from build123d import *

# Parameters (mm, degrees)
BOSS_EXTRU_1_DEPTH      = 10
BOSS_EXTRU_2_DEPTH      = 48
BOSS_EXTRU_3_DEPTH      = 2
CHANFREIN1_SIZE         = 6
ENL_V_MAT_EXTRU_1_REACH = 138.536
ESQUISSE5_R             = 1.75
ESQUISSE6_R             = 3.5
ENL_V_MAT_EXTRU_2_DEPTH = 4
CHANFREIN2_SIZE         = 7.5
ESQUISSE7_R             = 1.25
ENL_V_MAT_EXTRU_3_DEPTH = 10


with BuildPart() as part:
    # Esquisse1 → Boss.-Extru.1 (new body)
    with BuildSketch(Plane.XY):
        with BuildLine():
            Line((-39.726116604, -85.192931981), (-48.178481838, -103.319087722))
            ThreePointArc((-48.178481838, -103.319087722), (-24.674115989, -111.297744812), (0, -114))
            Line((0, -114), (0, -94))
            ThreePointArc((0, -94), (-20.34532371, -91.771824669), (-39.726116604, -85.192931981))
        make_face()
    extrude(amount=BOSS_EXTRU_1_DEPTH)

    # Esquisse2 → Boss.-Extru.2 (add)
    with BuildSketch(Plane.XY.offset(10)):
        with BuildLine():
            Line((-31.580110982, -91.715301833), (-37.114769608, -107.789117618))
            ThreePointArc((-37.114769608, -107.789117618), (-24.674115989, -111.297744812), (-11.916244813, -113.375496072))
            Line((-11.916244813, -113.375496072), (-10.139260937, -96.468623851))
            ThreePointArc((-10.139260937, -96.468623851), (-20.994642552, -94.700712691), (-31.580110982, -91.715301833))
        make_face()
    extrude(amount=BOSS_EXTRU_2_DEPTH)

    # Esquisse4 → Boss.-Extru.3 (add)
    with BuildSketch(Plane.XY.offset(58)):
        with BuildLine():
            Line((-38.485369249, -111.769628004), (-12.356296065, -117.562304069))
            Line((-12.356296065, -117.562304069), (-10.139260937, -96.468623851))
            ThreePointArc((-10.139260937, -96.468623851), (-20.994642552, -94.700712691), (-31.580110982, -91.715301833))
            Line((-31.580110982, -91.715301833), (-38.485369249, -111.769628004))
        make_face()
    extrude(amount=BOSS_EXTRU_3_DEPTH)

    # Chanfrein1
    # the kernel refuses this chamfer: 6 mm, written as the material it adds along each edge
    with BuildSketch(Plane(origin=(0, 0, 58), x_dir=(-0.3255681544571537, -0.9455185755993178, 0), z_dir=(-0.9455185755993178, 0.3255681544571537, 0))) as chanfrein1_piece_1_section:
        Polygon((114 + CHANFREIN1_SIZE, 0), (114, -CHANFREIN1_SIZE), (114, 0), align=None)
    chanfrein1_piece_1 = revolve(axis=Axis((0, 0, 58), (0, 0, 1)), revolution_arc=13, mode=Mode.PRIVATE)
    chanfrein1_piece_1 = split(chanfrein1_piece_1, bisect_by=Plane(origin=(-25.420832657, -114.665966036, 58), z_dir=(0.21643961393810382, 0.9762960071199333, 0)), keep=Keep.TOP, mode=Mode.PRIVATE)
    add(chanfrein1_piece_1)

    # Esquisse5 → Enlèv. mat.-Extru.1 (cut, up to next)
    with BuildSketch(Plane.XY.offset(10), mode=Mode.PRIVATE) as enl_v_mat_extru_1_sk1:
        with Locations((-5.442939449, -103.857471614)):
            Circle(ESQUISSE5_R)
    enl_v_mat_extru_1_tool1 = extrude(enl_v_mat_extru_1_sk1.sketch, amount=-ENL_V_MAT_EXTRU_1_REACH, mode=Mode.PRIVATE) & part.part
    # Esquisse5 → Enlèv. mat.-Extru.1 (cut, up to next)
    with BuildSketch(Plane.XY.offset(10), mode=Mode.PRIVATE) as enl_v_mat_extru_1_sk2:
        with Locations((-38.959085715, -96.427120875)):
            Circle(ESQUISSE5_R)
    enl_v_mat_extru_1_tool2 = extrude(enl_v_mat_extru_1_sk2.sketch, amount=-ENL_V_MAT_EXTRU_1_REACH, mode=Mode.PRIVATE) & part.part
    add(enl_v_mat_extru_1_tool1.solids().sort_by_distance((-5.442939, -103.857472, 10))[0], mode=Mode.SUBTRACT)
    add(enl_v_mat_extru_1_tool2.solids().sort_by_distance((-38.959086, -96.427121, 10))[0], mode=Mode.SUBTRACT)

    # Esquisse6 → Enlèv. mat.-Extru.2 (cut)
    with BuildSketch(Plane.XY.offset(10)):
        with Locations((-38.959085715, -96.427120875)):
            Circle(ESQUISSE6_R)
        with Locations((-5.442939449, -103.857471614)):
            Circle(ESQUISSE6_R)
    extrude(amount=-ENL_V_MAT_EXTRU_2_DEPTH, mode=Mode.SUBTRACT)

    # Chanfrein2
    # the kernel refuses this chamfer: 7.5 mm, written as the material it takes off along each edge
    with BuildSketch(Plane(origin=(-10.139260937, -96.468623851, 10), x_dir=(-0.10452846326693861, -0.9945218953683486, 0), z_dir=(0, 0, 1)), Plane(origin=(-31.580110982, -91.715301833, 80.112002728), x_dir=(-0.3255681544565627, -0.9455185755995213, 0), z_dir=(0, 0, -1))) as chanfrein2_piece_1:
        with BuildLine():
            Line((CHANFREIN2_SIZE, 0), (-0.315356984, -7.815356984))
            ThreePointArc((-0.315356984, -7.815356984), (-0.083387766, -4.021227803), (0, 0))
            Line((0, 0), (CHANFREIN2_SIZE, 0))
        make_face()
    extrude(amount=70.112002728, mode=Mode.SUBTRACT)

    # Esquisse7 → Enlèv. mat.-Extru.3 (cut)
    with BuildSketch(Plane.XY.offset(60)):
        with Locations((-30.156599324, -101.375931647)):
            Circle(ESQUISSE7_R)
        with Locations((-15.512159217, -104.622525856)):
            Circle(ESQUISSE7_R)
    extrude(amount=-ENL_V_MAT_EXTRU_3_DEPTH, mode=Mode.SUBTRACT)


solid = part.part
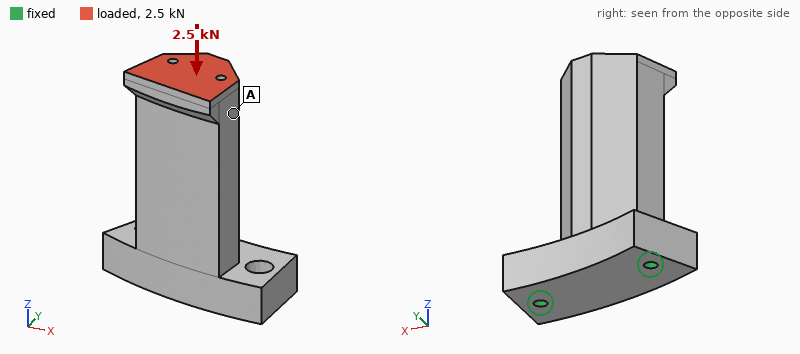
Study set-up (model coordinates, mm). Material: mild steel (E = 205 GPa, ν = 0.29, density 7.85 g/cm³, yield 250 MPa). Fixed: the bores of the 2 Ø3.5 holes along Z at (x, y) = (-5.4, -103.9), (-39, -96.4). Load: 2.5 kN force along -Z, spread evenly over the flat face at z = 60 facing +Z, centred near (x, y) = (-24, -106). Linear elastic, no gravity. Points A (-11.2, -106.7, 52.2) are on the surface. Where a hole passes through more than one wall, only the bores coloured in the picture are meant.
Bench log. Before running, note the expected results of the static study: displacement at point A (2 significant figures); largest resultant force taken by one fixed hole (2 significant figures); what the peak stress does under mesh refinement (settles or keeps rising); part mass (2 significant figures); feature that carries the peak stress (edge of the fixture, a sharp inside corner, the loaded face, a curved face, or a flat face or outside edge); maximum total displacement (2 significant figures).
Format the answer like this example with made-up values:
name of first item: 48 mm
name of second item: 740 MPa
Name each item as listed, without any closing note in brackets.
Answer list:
displacement at point A: 25 µm
largest resultant force taken by one fixed hole: 1.4 kN
what the peak stress does under mesh refinement: keeps rising
part mass: 210 g
feature that carries the peak stress: edge of the fixture
maximum total displacement: 32 µm
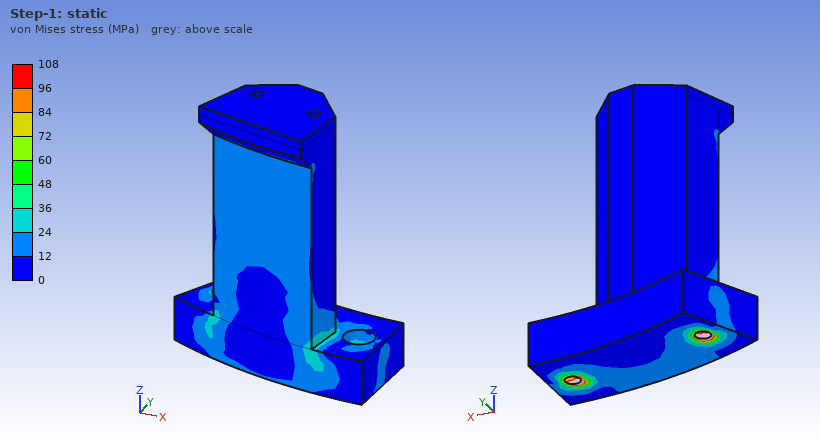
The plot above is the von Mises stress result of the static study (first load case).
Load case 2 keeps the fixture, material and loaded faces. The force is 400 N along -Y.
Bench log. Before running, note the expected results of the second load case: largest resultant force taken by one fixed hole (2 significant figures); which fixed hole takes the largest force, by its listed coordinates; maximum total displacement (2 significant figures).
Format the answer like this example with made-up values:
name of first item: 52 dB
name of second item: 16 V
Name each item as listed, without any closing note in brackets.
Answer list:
largest resultant force taken by one fixed hole: 290 N
which fixed hole takes the largest force, by its listed coordinates: (-39, -96.4)
maximum total displacement: 56 µm
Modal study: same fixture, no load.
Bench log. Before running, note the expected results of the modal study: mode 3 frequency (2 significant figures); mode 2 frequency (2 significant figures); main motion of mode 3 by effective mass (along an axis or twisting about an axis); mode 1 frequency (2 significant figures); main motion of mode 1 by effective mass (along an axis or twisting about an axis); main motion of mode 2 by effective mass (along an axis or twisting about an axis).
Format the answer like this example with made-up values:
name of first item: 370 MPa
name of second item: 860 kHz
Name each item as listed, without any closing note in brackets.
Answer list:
mode 3 frequency: 11 kHz
mode 2 frequency: 4400 Hz
main motion of mode 3 by effective mass: along Z
mode 1 frequency: 1900 Hz
main motion of mode 1 by effective mass: along Y
main motion of mode 2 by effective mass: along X
